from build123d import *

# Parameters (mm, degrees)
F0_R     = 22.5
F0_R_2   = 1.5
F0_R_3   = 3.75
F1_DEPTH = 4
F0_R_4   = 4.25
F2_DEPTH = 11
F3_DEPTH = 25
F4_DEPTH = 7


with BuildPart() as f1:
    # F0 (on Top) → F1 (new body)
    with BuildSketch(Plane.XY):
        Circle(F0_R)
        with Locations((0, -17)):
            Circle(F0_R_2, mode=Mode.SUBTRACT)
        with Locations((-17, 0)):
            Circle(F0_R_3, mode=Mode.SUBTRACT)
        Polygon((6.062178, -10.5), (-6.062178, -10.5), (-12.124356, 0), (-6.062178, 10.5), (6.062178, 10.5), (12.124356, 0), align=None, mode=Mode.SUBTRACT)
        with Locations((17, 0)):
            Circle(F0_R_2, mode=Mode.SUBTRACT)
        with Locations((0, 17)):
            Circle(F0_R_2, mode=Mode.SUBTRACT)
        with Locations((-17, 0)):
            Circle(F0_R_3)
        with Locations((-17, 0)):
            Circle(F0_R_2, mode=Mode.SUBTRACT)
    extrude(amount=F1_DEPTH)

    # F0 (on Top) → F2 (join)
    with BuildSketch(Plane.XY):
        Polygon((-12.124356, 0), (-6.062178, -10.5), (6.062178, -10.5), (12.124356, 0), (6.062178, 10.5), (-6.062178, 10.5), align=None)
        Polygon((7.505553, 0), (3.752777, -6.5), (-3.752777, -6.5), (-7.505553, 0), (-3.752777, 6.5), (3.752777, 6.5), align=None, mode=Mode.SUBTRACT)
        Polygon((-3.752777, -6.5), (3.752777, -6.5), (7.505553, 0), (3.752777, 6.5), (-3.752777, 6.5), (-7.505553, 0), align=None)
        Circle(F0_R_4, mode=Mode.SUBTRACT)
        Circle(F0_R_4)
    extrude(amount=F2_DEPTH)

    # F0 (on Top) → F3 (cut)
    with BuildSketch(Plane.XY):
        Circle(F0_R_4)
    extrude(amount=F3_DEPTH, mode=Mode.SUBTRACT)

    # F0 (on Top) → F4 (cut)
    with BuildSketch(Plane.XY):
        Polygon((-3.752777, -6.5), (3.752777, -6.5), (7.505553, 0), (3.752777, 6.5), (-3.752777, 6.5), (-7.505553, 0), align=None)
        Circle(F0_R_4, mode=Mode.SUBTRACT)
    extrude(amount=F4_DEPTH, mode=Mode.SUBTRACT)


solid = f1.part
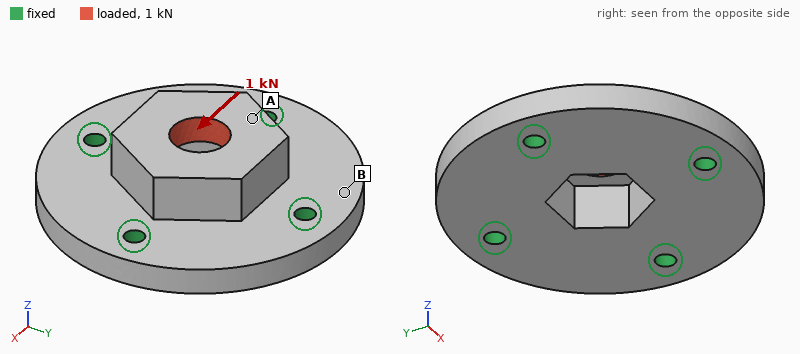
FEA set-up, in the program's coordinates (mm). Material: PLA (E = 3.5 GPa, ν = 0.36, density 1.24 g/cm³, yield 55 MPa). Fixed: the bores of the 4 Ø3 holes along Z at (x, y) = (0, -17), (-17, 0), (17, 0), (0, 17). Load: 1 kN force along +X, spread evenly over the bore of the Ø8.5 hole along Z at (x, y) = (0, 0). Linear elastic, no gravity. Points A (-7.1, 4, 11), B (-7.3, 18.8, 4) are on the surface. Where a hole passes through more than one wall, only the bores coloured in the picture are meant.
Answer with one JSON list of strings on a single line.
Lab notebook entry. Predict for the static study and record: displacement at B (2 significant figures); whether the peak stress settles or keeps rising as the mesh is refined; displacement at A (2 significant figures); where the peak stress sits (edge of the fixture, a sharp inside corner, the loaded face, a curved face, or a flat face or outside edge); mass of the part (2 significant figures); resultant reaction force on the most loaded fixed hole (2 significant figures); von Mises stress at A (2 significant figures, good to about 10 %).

["0.016 mm", "keeps rising", "0.089 mm", "edge of the fixture", "9.5 g", "380 N", "7.8 MPa"]
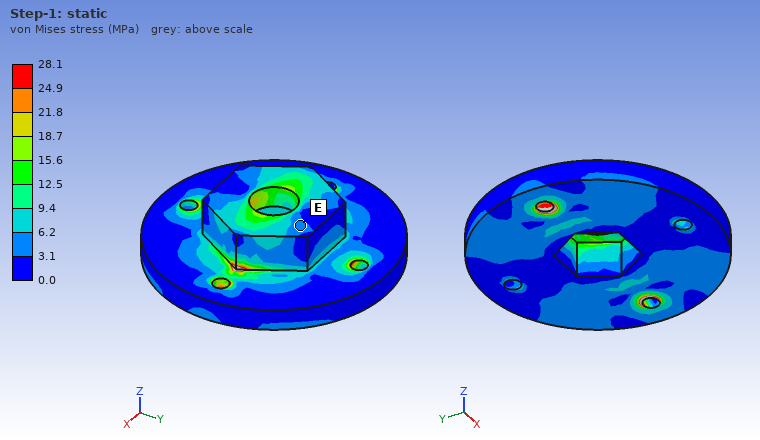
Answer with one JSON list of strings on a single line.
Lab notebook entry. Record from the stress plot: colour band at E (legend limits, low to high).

["3.1 to 6.2 MPa"]
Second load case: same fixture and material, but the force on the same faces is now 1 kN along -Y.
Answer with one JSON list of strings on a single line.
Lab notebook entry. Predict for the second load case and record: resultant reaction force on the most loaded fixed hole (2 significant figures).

["370 N"]
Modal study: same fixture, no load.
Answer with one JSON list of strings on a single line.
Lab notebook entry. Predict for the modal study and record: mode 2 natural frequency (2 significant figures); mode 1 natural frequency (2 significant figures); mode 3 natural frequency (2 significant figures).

["7800 Hz", "7700 Hz", "7800 Hz"]
